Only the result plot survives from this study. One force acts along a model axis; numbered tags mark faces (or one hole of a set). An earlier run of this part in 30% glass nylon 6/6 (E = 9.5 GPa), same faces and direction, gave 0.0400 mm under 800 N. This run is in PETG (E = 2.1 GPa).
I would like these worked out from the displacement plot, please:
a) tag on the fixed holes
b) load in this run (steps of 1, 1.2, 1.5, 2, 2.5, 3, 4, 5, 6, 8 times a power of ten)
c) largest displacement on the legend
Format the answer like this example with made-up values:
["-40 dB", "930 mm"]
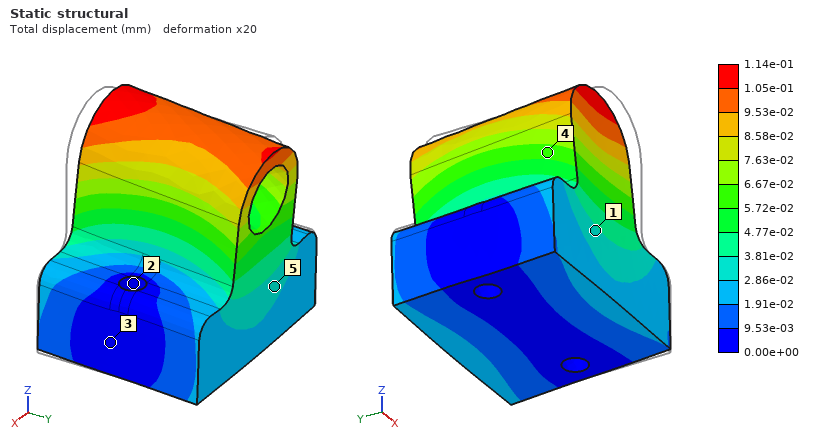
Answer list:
["2", "500 N", "1.14e-01 mm"]
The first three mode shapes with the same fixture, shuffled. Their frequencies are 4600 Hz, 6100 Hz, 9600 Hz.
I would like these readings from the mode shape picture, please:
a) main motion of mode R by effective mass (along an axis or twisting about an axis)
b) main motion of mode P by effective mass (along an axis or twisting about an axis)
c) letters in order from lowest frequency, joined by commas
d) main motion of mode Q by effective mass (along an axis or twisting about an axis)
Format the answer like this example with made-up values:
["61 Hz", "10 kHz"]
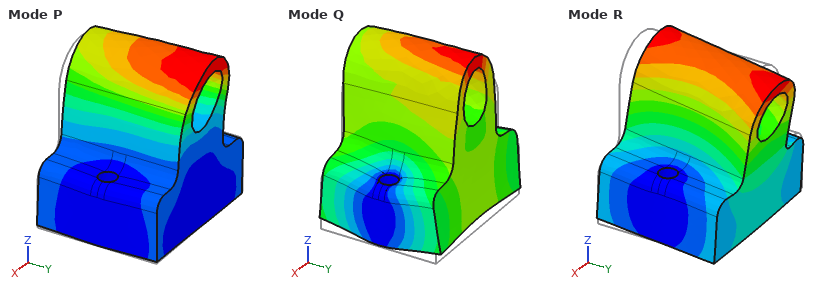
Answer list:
["along Y", "along X", "R, P, Q", "along Z"]
